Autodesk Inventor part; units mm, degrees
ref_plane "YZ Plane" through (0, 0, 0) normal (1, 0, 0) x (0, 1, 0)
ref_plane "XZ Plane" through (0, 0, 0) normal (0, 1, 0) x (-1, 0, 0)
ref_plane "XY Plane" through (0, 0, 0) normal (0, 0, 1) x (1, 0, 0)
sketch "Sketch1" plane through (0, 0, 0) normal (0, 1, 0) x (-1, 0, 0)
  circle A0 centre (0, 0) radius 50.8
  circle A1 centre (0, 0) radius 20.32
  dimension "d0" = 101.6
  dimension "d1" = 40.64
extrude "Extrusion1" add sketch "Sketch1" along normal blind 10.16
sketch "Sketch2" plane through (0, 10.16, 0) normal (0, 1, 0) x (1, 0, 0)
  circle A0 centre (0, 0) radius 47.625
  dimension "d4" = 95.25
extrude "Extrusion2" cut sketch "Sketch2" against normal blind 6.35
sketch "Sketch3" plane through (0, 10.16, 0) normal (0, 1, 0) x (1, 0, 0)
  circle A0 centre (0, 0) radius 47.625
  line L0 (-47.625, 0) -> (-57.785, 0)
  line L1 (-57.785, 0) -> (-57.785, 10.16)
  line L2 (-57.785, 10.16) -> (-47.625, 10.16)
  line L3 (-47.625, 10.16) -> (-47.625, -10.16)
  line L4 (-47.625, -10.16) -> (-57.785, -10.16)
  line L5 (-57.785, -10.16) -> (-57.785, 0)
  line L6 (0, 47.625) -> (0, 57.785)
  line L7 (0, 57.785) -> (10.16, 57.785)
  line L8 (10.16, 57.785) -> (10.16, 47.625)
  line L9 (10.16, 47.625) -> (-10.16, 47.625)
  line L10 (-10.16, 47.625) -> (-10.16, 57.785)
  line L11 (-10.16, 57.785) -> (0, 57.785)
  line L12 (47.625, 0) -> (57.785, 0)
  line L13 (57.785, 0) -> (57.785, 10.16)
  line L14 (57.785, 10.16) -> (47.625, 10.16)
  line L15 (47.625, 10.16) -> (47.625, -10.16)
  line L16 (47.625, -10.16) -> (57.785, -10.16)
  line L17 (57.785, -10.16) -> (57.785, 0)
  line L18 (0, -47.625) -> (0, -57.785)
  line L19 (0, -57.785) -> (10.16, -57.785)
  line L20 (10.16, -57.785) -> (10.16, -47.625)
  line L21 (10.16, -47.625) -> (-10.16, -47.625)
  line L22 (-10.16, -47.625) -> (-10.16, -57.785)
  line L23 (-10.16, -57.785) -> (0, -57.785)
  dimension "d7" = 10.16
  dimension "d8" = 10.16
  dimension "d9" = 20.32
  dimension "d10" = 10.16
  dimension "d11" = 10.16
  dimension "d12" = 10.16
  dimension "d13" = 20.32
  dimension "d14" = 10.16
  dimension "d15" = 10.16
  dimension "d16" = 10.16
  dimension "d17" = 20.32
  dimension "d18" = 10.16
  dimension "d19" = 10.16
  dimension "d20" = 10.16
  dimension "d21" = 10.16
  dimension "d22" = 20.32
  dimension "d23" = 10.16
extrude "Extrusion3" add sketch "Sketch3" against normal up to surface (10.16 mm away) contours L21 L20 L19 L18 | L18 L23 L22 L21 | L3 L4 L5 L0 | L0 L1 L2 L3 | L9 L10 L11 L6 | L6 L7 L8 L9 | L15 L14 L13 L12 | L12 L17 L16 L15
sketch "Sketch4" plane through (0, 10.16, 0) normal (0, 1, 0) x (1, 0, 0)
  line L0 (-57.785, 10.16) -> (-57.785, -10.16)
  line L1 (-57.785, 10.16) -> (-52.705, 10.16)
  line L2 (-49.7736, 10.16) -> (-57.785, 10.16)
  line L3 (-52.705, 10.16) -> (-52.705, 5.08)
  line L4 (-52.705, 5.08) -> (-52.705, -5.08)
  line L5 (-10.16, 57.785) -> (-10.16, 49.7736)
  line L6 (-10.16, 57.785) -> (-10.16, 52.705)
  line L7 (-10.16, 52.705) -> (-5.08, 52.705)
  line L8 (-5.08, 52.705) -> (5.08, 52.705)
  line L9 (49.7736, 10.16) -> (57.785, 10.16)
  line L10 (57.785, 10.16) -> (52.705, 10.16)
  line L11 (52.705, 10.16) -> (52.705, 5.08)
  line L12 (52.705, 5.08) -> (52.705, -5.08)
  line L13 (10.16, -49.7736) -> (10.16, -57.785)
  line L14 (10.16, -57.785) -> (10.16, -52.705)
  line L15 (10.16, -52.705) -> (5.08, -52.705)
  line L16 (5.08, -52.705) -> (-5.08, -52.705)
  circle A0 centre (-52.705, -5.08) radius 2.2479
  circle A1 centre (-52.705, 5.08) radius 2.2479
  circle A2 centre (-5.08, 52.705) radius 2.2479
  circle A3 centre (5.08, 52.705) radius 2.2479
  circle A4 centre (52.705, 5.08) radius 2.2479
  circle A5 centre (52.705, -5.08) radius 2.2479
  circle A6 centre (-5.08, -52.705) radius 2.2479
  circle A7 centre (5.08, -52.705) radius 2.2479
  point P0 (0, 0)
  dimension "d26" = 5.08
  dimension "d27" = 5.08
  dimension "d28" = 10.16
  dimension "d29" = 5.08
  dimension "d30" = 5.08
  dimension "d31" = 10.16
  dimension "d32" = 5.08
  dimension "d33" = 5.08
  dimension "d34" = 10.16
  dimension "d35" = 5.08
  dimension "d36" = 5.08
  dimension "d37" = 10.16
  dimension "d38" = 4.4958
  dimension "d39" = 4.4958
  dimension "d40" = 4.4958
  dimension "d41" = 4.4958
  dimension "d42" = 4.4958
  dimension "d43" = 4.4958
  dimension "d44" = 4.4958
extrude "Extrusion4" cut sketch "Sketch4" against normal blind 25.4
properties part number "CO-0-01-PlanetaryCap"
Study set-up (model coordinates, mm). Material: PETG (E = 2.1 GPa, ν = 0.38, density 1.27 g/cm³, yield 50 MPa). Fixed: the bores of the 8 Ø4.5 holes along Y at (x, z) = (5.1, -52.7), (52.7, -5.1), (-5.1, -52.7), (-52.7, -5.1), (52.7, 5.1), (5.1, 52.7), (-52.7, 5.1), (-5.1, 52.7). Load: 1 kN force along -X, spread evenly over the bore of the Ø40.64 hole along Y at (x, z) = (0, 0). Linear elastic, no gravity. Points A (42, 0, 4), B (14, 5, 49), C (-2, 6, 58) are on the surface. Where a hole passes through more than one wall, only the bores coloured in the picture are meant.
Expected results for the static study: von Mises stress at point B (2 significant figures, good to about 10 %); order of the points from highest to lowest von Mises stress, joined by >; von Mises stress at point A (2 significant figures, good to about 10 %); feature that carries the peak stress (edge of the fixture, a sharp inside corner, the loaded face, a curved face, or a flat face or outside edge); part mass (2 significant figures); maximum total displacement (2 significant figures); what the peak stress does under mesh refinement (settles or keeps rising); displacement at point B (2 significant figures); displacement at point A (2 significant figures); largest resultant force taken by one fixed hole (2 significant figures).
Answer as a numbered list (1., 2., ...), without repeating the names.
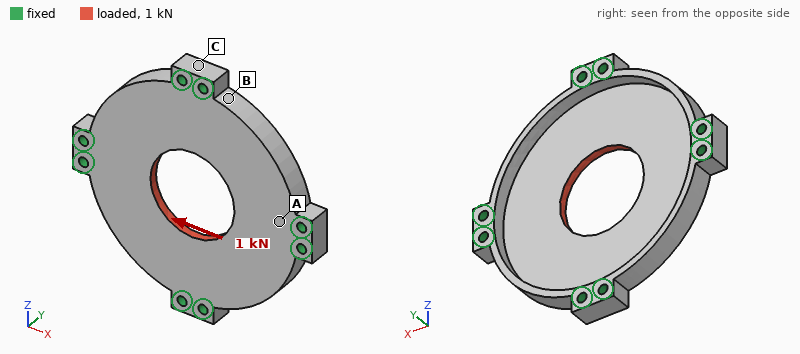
1. 1.5 MPa
2. A > B > C
3. 3.6 MPa
4. edge of the fixture
5. 47 g
6. 66 µm
7. keeps rising
8. 12 µm
9. 21 µm
10. 170 N
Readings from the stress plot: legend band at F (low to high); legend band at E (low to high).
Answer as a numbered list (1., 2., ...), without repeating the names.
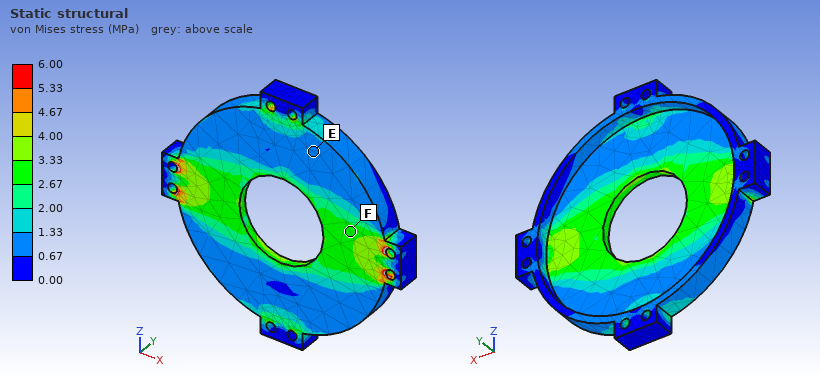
1. 2.67 to 3.33 MPa
2. 0.67 to 1.33 MPa
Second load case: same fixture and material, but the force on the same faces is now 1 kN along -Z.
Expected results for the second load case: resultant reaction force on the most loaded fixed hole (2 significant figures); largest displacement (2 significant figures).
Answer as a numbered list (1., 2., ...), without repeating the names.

1. 170 N
2. 66 µm
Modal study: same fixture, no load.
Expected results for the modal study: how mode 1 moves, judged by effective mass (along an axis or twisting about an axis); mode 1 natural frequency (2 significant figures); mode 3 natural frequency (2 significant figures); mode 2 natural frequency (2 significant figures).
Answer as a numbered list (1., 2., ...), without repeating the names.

1. along Y
2. 1000 Hz
3. 1500 Hz
4. 1500 Hz
